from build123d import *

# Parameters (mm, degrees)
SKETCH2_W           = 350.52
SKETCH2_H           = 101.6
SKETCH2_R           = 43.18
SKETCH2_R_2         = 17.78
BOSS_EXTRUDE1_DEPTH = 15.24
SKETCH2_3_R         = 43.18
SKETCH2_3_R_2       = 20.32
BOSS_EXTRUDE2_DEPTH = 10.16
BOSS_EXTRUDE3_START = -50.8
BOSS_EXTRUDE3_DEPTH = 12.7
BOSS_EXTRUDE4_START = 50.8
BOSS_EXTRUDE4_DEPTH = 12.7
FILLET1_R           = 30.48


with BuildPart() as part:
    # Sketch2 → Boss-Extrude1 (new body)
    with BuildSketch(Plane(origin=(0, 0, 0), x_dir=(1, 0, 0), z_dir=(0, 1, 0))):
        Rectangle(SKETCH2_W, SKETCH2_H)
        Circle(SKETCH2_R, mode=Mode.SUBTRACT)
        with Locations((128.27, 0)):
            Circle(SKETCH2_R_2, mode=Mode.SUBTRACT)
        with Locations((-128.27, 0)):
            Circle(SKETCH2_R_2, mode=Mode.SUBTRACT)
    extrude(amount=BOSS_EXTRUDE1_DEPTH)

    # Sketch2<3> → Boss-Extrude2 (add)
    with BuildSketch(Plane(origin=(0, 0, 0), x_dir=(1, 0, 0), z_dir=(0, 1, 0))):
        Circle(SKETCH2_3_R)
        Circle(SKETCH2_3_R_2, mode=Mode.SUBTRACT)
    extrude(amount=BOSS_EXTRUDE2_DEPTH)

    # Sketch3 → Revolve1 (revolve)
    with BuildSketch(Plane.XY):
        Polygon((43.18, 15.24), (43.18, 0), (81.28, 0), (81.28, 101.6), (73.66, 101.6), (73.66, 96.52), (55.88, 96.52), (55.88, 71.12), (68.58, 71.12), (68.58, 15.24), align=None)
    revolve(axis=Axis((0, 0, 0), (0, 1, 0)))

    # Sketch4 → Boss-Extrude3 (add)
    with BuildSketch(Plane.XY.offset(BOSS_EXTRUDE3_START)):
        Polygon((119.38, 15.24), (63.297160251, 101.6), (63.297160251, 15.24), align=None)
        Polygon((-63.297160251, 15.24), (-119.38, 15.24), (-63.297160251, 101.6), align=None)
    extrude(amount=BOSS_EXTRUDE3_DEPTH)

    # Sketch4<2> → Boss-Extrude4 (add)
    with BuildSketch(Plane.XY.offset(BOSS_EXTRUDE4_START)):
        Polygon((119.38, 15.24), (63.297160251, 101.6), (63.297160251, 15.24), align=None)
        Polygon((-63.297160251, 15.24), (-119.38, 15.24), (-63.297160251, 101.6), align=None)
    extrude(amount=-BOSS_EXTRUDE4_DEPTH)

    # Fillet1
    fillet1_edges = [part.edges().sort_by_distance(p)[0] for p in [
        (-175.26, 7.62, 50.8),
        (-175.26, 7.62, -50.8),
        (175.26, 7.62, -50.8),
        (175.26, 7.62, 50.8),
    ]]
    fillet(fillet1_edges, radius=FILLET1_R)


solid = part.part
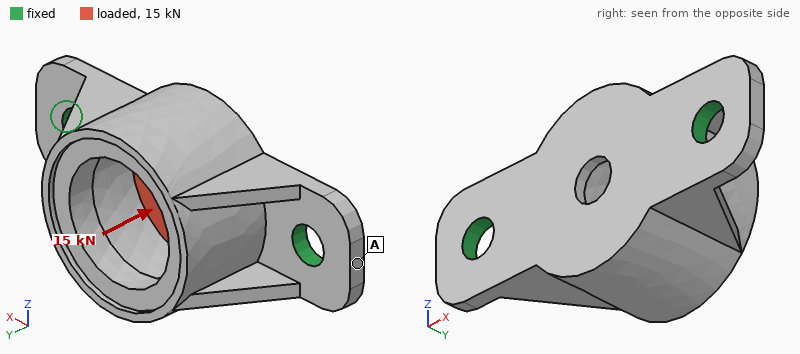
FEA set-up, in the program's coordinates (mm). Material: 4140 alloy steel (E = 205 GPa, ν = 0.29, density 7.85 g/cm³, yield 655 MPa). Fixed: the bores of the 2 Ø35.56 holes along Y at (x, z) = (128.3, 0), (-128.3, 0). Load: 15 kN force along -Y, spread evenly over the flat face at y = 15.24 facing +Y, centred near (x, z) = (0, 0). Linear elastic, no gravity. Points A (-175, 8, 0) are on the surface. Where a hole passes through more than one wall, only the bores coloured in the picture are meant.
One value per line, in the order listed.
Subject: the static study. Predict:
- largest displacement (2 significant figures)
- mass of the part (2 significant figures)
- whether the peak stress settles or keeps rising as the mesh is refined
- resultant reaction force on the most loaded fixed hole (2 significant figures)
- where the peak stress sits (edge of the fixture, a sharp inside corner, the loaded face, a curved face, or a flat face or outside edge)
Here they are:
23 µm
10 kg
keeps rising
8.4 kN
edge of the fixture
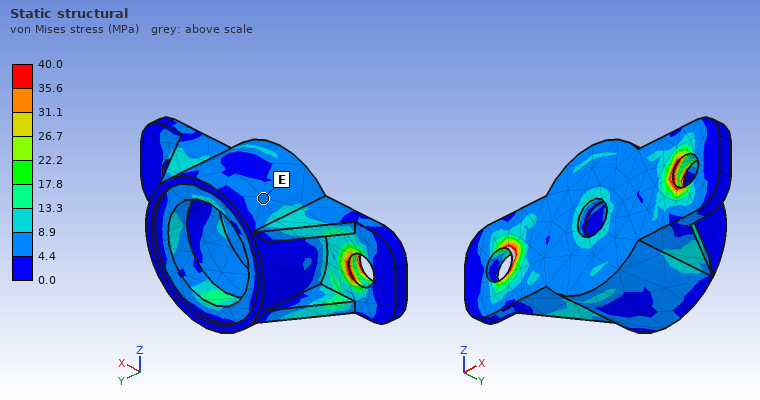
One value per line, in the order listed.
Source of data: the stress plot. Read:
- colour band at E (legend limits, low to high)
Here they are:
4.4 to 8.9 MPa
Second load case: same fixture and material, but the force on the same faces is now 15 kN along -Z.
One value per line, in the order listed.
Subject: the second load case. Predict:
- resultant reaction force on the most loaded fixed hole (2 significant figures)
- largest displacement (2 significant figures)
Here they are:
7.5 kN
18 µm
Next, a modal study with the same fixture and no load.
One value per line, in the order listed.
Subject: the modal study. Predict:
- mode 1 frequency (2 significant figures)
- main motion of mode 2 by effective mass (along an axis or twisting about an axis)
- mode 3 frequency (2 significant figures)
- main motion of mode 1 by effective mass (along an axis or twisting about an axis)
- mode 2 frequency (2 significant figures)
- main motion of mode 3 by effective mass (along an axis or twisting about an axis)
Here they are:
920 Hz
along Y
3100 Hz
along Z
1800 Hz
along X
